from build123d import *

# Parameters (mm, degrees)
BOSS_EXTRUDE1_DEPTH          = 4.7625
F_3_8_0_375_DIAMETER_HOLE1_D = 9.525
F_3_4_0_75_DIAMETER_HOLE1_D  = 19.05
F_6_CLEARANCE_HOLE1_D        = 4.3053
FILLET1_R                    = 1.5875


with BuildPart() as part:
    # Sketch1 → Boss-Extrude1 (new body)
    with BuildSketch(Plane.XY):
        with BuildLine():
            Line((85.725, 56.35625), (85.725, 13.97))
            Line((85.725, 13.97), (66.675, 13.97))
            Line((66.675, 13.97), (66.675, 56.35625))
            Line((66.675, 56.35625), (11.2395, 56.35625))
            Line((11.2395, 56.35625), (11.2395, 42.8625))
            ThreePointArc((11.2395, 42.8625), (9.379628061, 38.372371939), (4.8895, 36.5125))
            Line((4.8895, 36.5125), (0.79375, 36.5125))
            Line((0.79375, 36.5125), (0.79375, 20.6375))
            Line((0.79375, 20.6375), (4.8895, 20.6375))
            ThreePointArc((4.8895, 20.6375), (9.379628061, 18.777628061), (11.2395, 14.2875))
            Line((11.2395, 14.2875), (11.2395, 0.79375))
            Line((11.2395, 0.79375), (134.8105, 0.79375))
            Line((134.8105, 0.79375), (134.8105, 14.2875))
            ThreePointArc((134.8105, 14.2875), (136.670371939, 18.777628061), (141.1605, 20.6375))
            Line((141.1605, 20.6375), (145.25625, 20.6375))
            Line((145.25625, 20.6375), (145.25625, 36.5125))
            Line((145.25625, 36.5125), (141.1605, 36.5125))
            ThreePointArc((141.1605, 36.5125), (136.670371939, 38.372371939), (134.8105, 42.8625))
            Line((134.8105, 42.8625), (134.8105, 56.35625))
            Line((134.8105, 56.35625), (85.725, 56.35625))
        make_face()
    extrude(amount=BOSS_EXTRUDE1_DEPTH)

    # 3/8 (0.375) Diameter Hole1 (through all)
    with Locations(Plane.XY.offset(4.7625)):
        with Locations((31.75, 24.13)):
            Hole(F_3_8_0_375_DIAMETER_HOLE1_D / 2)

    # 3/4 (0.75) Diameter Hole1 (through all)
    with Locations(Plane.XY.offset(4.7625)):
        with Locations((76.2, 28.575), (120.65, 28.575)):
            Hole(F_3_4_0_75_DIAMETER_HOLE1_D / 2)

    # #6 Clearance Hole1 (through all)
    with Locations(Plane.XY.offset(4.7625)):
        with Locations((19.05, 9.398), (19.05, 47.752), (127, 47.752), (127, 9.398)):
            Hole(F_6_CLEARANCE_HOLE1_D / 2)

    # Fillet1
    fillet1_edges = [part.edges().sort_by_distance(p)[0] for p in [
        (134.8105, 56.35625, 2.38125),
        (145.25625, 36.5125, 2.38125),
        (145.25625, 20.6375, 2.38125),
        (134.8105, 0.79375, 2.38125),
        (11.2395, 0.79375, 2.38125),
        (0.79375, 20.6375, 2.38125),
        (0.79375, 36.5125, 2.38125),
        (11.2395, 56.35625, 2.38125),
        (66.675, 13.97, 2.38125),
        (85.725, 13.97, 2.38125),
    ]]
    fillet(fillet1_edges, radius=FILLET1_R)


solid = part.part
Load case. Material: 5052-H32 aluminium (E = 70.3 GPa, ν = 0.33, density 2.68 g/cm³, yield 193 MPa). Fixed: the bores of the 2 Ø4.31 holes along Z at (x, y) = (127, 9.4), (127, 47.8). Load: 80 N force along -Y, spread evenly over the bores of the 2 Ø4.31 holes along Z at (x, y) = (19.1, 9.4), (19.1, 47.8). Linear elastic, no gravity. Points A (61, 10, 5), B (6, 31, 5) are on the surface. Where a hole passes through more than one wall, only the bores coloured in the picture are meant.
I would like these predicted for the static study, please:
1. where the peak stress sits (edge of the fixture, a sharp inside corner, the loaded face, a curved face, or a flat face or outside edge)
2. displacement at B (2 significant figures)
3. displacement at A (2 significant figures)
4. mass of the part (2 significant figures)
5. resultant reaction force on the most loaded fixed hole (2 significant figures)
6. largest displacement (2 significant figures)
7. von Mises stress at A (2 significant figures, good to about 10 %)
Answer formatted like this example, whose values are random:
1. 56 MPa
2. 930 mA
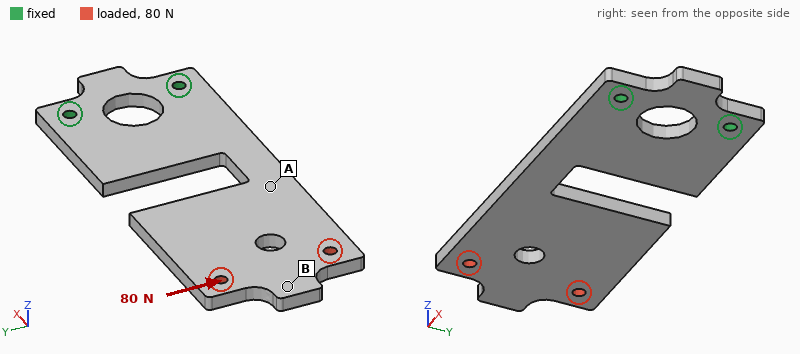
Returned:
1. a curved face
2. 0.19 mm
3. 0.046 mm
4. 77 g
5. 230 N
6. 0.21 mm
7. 8.2 MPa
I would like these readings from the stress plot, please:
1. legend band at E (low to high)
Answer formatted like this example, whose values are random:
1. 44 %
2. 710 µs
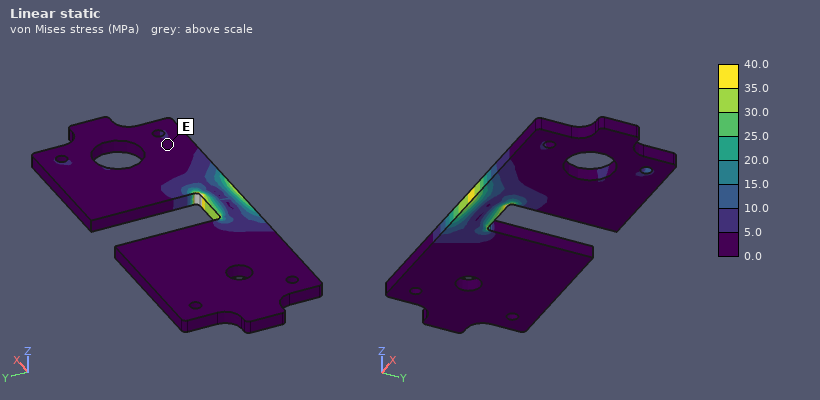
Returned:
1. 0.0 to 5.0 MPa
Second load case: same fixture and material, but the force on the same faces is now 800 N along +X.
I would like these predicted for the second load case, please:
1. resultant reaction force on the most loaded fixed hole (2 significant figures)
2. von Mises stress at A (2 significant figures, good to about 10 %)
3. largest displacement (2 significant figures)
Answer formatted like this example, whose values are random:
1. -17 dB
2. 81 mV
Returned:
1. 440 N
2. 37 MPa
3. 0.70 mm
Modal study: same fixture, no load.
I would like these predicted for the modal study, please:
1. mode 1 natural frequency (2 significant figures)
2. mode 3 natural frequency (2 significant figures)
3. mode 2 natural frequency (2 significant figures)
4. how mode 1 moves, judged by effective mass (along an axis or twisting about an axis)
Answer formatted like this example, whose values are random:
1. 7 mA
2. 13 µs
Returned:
1. 190 Hz
2. 690 Hz
3. 670 Hz
4. along Z
